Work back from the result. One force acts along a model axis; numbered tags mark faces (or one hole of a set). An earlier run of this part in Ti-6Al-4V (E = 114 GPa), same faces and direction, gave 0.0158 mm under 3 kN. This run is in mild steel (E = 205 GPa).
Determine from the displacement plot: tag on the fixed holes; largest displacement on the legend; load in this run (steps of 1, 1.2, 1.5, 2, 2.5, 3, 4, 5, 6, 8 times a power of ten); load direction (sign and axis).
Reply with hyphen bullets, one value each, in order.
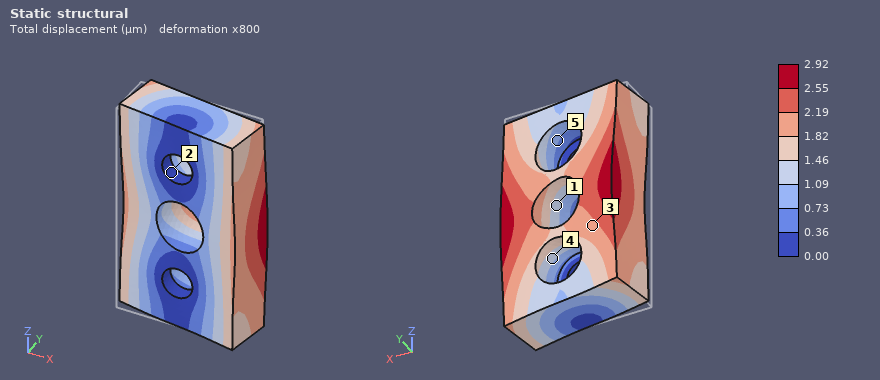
- 2
- 2.92 µm
- 1 kN
- +X
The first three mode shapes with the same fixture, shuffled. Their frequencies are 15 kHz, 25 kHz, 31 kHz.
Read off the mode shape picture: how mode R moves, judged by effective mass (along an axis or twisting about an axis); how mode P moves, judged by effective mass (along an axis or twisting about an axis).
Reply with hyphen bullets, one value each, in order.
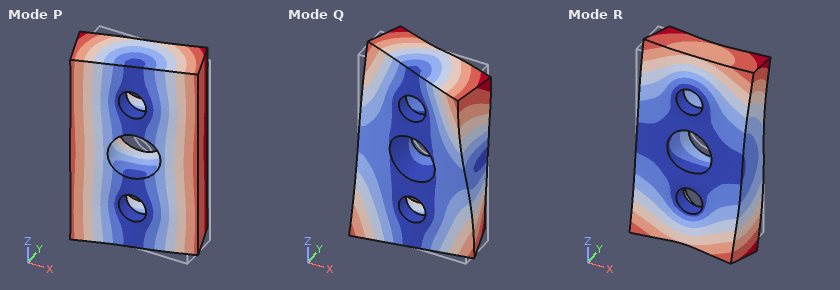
- along Z
- along X
